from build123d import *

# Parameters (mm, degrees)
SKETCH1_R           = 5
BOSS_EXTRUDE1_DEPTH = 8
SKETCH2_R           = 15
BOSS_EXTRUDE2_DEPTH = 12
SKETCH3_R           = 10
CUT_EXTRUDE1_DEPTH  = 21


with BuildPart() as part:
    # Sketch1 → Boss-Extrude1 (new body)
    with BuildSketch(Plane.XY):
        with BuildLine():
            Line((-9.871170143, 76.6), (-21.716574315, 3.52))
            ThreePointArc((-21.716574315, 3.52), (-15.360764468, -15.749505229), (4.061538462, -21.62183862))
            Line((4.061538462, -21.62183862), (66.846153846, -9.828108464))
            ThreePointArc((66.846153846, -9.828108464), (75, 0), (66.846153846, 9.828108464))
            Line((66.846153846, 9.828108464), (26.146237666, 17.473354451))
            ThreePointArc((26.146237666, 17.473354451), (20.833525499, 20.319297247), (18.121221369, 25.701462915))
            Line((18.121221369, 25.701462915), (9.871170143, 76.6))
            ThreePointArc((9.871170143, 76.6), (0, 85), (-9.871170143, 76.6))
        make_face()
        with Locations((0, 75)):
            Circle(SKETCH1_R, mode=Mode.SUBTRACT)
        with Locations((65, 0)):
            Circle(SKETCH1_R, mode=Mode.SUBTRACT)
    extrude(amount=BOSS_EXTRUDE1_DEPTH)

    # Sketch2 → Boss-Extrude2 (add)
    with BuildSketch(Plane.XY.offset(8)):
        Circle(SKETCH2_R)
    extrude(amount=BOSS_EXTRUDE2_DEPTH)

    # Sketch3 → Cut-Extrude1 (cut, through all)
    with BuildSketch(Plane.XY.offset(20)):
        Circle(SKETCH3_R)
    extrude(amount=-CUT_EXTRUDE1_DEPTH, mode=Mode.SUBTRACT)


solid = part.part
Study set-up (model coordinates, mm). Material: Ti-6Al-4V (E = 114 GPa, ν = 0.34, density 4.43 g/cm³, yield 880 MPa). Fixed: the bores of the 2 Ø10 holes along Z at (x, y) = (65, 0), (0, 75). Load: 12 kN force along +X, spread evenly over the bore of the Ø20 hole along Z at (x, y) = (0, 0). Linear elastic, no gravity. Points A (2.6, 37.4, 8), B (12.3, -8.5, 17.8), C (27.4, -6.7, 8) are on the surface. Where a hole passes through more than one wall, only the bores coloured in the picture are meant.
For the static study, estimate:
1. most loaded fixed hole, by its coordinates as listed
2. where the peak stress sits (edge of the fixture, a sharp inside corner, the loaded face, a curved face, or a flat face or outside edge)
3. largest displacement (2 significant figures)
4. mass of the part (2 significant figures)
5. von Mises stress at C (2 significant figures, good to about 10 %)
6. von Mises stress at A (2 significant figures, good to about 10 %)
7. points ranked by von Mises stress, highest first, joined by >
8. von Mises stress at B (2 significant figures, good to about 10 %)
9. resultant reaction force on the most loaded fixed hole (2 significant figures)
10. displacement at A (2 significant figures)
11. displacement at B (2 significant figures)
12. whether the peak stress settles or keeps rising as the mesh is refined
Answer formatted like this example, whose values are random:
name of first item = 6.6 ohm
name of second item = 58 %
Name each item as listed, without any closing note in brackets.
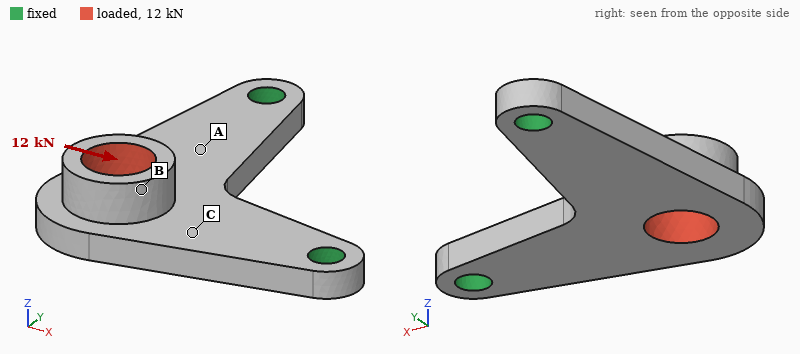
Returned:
most loaded fixed hole, by its coordinates as listed = (65, 0)
where the peak stress sits = edge of the fixture
largest displacement = 0.52 mm
mass of the part = 180 g
von Mises stress at C = 130 MPa
von Mises stress at A = 81 MPa
points ranked by von Mises stress, highest first, joined by > = C > A > B
von Mises stress at B = 26 MPa
resultant reaction force on the most loaded fixed hole = 12 kN
displacement at A = 0.10 mm
displacement at B = 0.27 mm
whether the peak stress settles or keeps rising as the mesh is refined = keeps rising
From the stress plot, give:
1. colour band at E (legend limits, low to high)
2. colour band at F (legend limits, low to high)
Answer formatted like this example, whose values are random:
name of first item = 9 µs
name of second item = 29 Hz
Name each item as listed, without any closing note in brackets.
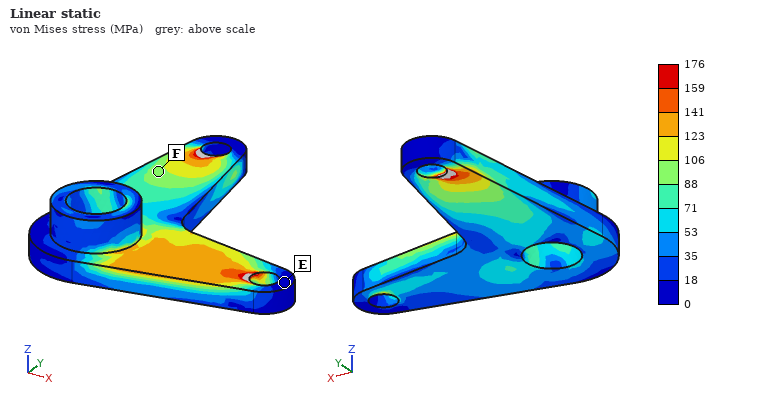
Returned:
colour band at E = 0 to 18 MPa
colour band at F = 88 to 106 MPa
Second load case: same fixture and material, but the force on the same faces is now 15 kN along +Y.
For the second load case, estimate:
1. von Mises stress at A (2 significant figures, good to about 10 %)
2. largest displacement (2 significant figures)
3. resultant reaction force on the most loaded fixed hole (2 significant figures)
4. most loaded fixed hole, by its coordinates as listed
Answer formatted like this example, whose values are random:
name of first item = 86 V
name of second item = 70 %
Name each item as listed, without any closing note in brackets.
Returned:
von Mises stress at A = 130 MPa
largest displacement = 0.55 mm
resultant reaction force on the most loaded fixed hole = 14 kN
most loaded fixed hole, by its coordinates as listed = (0, 75)
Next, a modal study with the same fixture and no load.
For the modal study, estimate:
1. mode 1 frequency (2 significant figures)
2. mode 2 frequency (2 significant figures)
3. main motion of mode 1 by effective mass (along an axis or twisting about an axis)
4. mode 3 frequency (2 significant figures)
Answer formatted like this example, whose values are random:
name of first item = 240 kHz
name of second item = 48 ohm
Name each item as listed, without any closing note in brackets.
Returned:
mode 1 frequency = 1200 Hz
mode 2 frequency = 4400 Hz
main motion of mode 1 by effective mass = along Z
mode 3 frequency = 5200 Hz
